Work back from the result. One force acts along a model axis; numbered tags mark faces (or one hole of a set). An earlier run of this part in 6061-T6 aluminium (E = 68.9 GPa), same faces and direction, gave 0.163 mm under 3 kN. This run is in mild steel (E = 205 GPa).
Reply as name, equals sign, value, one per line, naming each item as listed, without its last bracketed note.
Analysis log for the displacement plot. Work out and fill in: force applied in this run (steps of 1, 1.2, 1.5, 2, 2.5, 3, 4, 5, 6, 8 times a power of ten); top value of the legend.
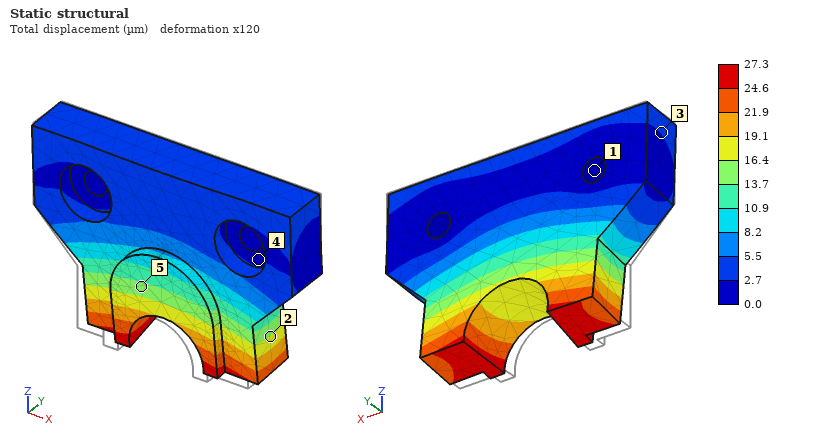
force applied in this run = 1.5 kN
top value of the legend = 27.3 µm
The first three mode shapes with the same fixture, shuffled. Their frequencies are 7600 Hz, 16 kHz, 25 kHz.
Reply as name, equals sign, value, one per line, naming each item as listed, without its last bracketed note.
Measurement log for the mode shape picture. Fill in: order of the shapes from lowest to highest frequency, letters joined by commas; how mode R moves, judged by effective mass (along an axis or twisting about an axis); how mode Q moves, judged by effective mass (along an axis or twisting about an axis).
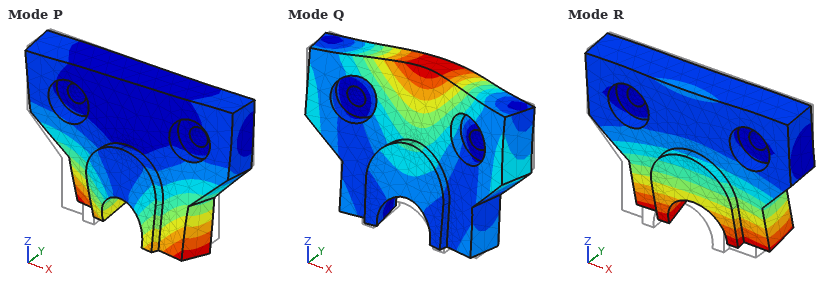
order of the shapes from lowest to highest frequency, letters joined by commas = R, P, Q
how mode R moves, judged by effective mass = along Y
how mode Q moves, judged by effective mass = along Y
